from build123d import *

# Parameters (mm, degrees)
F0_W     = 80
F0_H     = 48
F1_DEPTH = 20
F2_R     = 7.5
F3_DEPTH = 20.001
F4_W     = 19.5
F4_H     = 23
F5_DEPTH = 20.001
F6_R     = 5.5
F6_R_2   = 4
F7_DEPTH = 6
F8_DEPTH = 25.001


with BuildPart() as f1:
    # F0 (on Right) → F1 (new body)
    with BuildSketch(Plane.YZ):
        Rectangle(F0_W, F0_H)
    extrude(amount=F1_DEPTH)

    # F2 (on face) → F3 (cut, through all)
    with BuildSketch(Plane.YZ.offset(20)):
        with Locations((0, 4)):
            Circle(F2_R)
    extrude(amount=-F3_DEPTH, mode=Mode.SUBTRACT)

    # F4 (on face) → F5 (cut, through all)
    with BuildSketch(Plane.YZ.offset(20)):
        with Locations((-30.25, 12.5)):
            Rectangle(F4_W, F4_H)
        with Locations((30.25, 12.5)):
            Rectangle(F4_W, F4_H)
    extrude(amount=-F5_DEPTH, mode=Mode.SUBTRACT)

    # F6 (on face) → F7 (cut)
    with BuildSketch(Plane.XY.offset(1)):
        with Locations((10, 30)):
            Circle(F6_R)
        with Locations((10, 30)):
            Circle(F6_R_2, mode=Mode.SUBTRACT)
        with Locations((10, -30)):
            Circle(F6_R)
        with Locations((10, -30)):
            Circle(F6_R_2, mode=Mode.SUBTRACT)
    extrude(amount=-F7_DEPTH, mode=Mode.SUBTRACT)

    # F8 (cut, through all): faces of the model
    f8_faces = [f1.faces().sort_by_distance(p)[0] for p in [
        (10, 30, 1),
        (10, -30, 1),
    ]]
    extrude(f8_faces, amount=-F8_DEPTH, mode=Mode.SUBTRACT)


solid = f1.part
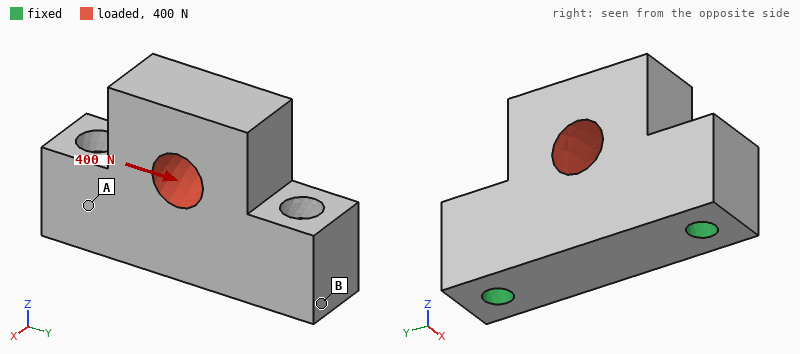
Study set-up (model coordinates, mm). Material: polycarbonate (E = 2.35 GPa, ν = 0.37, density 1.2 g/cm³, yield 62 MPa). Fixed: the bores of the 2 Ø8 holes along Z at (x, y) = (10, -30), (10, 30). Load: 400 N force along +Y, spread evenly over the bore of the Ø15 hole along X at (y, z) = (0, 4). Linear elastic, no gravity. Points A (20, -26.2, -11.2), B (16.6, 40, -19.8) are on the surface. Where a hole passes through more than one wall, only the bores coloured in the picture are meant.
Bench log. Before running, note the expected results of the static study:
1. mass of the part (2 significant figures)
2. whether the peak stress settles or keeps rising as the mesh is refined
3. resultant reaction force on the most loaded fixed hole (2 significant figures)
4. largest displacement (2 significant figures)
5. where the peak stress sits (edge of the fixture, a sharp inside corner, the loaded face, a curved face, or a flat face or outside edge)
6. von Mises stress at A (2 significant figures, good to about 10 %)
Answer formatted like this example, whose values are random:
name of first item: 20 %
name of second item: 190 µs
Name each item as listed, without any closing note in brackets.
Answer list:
mass of the part: 63 g
whether the peak stress settles or keeps rising as the mesh is refined: keeps rising
resultant reaction force on the most loaded fixed hole: 230 N
largest displacement: 17 µm
where the peak stress sits: a sharp inside corner
von Mises stress at A: 0.38 MPa
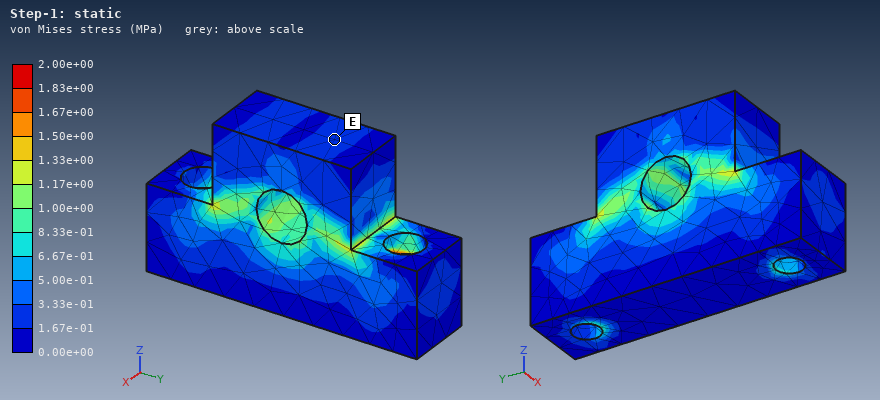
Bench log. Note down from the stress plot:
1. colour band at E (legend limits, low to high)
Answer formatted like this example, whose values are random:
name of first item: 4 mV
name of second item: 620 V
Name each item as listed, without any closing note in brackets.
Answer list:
colour band at E: 1.67e-01 to 3.33e-01 MPa
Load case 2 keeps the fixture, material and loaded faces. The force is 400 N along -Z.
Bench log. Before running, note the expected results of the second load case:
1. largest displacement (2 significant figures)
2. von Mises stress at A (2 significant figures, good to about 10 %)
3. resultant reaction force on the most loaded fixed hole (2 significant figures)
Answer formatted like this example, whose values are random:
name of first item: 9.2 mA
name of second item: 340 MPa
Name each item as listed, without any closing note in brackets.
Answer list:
largest displacement: 15 µm
von Mises stress at A: 0.58 MPa
resultant reaction force on the most loaded fixed hole: 210 N
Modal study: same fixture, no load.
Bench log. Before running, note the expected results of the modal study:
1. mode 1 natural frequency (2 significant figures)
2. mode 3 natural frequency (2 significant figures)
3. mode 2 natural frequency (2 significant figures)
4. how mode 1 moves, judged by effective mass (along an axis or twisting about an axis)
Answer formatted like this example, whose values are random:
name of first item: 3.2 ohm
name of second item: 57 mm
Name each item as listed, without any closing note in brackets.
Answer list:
mode 1 natural frequency: 1900 Hz
mode 3 natural frequency: 4300 Hz
mode 2 natural frequency: 4300 Hz
how mode 1 moves, judged by effective mass: along X
